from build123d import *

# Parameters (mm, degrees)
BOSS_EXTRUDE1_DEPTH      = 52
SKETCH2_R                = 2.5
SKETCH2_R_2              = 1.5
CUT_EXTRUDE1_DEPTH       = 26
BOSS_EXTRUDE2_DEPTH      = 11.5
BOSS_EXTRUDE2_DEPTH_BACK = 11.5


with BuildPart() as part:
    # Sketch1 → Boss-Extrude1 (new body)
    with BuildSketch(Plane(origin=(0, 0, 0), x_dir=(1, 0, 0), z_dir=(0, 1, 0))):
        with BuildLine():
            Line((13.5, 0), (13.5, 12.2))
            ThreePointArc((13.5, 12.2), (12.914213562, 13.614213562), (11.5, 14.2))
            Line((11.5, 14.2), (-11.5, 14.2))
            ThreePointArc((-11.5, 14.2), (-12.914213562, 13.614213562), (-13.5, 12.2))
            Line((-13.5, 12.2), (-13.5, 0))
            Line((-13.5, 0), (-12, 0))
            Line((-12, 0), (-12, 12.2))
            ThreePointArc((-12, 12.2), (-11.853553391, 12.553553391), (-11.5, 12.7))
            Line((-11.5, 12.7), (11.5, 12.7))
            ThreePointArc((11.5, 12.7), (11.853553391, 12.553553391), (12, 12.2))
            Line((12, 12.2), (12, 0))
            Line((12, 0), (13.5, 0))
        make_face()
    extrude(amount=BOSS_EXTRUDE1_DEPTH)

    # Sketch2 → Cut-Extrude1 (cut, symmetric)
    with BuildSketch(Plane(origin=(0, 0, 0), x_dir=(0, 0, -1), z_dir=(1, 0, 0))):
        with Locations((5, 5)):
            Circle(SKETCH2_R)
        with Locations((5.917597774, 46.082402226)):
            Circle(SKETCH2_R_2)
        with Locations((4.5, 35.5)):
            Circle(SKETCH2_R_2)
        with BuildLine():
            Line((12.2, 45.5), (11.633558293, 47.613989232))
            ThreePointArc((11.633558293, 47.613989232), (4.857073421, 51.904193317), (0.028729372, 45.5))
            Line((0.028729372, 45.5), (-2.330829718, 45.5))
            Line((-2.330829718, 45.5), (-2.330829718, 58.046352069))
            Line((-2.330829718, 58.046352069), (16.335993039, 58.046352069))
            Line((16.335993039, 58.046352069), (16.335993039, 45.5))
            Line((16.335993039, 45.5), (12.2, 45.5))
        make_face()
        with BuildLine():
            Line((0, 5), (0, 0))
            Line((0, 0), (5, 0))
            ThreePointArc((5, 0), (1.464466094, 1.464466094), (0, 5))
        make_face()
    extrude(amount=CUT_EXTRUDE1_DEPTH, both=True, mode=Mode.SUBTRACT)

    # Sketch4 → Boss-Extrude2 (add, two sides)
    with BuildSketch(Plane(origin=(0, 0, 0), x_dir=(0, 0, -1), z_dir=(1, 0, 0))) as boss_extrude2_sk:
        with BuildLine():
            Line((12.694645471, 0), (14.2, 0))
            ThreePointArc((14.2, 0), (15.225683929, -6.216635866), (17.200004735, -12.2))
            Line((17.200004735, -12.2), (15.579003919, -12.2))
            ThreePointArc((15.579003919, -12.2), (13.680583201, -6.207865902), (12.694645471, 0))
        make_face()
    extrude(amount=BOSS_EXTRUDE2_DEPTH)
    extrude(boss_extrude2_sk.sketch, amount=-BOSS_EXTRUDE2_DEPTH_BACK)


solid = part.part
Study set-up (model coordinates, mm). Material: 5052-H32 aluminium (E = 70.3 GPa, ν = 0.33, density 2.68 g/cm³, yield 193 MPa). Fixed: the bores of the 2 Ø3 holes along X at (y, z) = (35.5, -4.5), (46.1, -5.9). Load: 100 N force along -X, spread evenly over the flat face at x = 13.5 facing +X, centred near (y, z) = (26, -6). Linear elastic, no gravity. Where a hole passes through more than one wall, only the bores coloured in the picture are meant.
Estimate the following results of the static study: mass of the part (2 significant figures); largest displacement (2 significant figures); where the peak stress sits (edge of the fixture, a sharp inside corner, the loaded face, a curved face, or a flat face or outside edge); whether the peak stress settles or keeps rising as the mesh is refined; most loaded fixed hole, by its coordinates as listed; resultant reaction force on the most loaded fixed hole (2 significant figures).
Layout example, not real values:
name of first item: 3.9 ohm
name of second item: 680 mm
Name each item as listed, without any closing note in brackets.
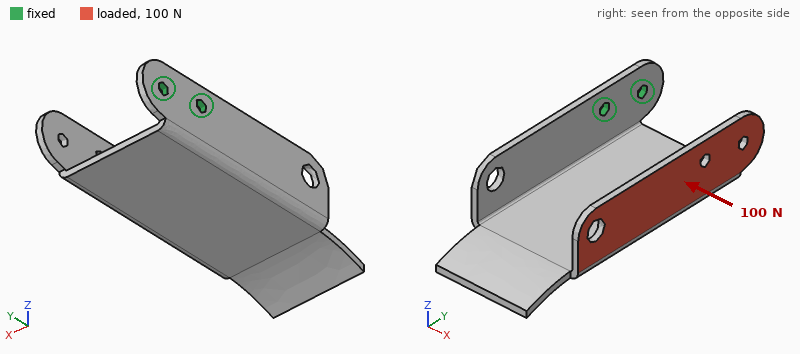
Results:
mass of the part: 11 g
largest displacement: 0.54 mm
where the peak stress sits: a sharp inside corner
whether the peak stress settles or keeps rising as the mesh is refined: keeps rising
most loaded fixed hole, by its coordinates as listed: (35.5, -4.5)
resultant reaction force on the most loaded fixed hole: 150 N
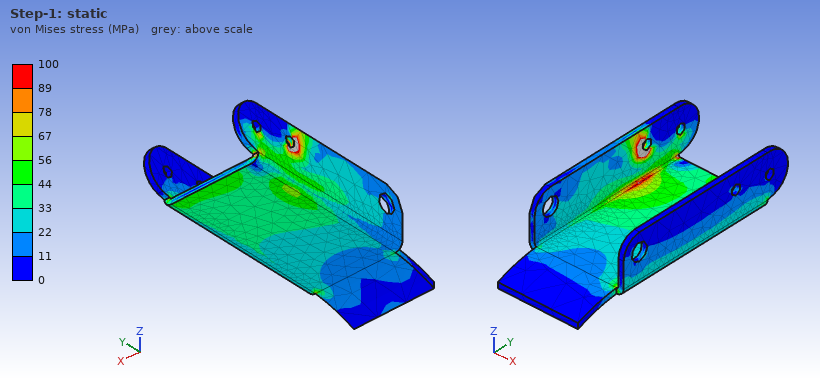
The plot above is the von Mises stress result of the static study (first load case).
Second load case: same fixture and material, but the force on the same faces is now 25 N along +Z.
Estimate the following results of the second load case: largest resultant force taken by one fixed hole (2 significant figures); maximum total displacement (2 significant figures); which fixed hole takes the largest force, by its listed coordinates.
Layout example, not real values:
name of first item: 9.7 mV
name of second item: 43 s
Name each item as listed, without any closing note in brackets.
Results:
largest resultant force taken by one fixed hole: 40 N
maximum total displacement: 0.53 mm
which fixed hole takes the largest force, by its listed coordinates: (35.5, -4.5)
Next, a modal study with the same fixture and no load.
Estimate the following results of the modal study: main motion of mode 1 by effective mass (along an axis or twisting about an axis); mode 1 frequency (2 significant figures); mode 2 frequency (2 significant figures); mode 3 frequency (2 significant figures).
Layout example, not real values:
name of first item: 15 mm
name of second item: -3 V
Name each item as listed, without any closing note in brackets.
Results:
main motion of mode 1 by effective mass: along Z
mode 1 frequency: 520 Hz
mode 2 frequency: 870 Hz
mode 3 frequency: 1300 Hz
